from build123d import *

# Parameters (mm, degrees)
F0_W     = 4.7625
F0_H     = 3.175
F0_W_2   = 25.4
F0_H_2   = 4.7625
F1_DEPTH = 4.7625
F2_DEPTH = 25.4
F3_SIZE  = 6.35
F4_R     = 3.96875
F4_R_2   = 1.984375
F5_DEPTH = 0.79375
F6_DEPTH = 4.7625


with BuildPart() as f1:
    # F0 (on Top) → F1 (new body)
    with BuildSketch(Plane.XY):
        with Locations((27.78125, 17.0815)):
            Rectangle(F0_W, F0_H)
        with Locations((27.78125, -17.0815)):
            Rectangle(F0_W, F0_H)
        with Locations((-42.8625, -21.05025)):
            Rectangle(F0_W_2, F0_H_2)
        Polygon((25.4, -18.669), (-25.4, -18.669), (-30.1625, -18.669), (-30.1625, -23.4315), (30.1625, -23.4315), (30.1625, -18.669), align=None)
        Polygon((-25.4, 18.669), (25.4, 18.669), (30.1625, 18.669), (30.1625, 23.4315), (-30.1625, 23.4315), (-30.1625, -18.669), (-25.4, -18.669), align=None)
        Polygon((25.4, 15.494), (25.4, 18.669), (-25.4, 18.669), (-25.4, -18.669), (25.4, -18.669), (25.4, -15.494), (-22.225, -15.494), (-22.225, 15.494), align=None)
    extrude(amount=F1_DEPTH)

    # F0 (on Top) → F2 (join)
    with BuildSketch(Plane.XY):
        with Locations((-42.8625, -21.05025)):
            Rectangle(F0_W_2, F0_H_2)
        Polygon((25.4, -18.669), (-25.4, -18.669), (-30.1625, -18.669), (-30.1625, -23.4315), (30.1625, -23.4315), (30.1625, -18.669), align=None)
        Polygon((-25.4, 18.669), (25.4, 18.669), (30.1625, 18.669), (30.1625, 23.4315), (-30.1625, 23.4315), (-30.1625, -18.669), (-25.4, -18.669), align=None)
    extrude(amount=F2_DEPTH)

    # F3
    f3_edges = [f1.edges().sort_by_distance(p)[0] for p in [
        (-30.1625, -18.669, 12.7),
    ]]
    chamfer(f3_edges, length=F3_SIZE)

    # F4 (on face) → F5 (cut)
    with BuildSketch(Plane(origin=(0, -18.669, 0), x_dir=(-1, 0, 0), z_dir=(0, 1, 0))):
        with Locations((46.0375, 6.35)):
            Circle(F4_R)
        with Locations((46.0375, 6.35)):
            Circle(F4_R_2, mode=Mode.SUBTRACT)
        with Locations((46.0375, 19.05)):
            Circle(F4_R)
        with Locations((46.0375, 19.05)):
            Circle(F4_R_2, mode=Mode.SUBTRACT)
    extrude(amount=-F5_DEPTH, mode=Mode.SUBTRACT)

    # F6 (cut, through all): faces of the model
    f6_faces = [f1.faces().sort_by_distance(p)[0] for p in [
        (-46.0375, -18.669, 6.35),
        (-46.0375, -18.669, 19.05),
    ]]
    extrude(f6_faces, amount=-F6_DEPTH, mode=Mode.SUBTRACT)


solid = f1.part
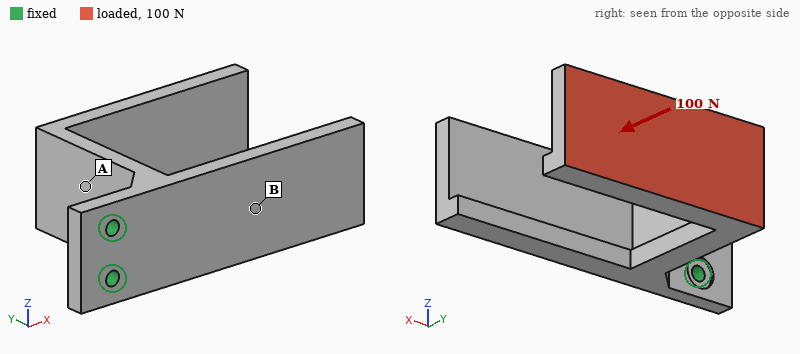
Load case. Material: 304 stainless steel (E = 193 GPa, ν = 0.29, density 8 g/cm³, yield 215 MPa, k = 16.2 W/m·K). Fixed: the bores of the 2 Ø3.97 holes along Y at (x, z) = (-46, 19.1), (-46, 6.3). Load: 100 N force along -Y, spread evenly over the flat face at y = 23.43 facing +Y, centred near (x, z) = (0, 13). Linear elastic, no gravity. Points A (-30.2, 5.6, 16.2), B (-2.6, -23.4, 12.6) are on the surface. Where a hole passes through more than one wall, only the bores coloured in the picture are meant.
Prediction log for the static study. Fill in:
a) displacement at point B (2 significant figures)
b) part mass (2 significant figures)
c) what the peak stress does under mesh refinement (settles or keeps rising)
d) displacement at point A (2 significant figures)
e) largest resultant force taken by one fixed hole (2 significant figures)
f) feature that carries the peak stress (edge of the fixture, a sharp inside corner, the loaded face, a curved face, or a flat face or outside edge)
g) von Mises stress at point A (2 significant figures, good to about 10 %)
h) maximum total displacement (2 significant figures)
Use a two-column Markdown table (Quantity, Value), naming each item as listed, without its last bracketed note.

| Quantity | Value |
|---|---|
| displacement at point B | 0.045 mm |
| part mass | 200 g |
| what the peak stress does under mesh refinement | keeps rising |
| displacement at point A | 0.041 mm |
| largest resultant force taken by one fixed hole | 51 N |
| feature that carries the peak stress | edge of the fixture |
| von Mises stress at point A | 15 MPa |
| maximum total displacement | 0.20 mm |
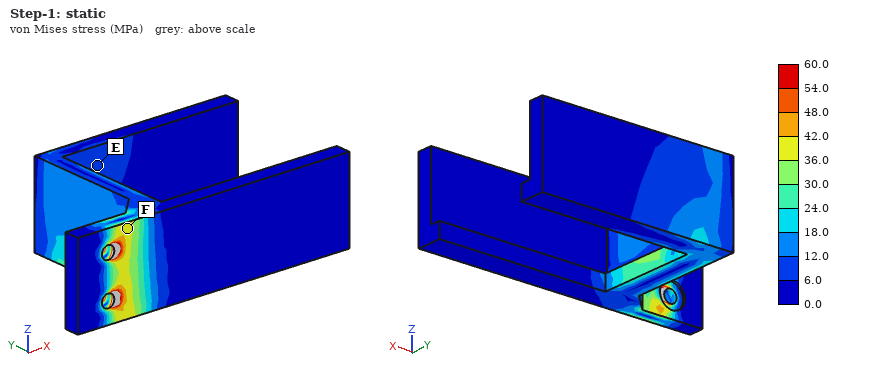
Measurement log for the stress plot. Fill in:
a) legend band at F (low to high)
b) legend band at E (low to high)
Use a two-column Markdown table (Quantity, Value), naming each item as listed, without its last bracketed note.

| Quantity | Value |
|---|---|
| legend band at F | 36.0 to 42.0 MPa |
| legend band at E | 6.0 to 12.0 MPa |
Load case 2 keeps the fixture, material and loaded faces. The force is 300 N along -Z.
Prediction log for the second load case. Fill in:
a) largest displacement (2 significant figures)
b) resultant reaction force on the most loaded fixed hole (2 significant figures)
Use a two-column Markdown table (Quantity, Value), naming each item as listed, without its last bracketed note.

| Quantity | Value |
|---|---|
| largest displacement | 0.22 mm |
| resultant reaction force on the most loaded fixed hole | 1.2 kN |
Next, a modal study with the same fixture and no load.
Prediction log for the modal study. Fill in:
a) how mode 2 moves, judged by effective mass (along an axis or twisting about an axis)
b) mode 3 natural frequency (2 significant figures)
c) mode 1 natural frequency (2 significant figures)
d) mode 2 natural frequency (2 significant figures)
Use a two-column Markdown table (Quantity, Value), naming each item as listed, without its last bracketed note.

| Quantity | Value |
|---|---|
| how mode 2 moves, judged by effective mass | along Z |
| mode 3 natural frequency | 1000 Hz |
| mode 1 natural frequency | 410 Hz |
| mode 2 natural frequency | 850 Hz |
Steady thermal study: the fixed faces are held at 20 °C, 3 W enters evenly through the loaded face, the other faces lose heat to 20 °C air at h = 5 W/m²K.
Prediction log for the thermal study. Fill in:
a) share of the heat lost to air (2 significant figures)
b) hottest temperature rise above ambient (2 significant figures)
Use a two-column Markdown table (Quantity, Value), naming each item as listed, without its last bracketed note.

| Quantity | Value |
|---|---|
| share of the heat lost to air | 46 % |
| hottest temperature rise above ambient | 71 K |
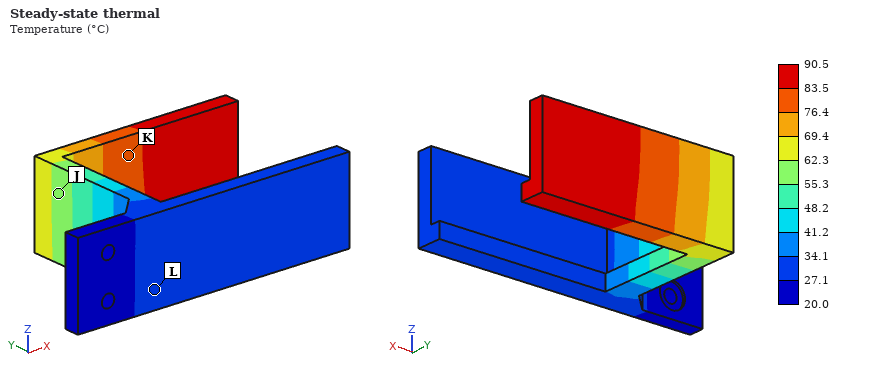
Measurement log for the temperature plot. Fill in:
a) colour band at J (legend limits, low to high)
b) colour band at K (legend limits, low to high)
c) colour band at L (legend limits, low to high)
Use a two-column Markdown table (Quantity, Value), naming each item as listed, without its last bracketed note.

| Quantity | Value |
|---|---|
| colour band at J | 55.3 to 62.3 °C |
| colour band at K | 76.4 to 83.5 °C |
| colour band at L | 27.1 to 34.1 °C |
